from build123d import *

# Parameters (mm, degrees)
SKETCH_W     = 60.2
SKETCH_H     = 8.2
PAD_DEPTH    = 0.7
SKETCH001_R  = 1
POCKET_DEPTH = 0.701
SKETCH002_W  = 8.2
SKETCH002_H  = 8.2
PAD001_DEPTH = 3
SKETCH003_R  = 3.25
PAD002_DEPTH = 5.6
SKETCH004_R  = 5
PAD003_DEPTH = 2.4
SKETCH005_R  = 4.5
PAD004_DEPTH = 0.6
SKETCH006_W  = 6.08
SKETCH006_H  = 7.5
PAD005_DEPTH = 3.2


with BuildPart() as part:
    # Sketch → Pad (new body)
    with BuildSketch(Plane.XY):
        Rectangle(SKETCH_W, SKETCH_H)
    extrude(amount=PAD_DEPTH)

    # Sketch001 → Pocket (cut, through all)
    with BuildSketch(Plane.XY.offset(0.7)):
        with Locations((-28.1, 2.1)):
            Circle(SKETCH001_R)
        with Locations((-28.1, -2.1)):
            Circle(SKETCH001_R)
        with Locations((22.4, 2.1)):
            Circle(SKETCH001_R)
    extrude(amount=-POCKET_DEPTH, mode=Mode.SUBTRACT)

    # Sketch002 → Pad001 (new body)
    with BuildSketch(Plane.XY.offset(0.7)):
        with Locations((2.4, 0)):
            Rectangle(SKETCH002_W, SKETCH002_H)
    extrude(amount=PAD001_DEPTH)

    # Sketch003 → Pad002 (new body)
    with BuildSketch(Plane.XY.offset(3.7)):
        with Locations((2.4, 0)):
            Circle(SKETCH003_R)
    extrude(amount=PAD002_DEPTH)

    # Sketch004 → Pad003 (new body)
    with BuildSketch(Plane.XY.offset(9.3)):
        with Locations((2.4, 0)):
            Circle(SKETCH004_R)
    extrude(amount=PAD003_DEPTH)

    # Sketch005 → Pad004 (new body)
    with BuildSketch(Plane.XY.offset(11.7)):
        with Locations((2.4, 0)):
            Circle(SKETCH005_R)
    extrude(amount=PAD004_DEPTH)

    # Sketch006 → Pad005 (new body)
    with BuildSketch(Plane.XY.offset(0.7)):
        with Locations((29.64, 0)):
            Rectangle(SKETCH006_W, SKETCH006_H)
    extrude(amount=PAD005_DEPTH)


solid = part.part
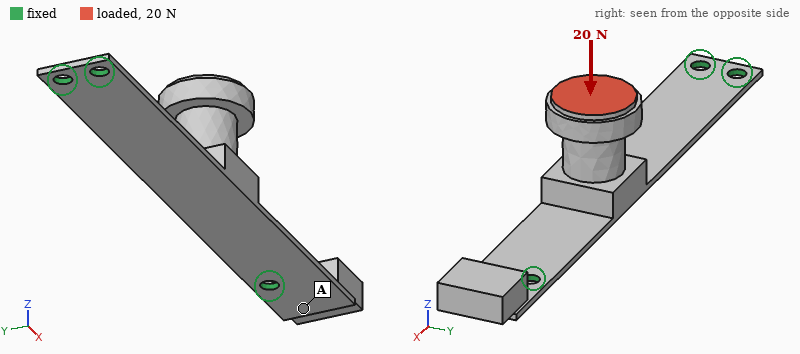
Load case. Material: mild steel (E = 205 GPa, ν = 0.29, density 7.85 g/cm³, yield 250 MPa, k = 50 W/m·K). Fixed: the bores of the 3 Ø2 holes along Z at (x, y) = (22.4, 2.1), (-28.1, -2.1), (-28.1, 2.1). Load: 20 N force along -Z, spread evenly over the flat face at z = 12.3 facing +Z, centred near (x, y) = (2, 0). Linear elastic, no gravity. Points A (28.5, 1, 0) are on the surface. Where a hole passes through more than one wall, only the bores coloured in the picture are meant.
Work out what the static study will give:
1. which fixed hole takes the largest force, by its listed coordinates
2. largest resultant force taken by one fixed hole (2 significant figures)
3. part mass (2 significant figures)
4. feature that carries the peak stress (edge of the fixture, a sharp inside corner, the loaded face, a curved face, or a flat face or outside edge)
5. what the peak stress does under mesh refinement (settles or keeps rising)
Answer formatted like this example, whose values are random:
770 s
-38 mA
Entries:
(22.4, 2.1)
15 N
8.6 g
edge of the fixture
keeps rising
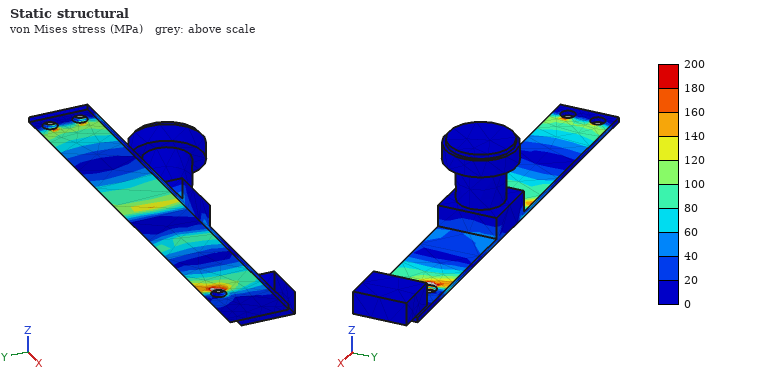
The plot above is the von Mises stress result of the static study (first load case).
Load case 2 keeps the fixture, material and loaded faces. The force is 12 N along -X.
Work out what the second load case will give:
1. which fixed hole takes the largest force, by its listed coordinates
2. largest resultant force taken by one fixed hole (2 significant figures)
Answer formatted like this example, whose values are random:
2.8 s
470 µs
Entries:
(22.4, 2.1)
7.1 N
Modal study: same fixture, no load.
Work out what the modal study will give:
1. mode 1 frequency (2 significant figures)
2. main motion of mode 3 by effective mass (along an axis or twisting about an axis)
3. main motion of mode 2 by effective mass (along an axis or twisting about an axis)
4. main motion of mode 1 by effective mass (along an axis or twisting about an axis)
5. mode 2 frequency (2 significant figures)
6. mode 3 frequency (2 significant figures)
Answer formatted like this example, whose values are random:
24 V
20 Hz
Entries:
760 Hz
along X
along Y
along Z
860 Hz
1800 Hz
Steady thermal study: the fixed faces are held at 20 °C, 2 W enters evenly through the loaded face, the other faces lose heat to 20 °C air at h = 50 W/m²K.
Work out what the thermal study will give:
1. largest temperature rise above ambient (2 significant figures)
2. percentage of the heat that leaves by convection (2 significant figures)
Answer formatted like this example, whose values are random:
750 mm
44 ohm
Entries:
40 K
67 %
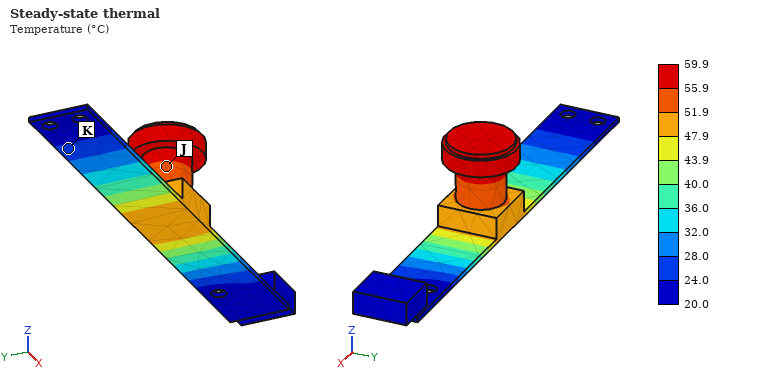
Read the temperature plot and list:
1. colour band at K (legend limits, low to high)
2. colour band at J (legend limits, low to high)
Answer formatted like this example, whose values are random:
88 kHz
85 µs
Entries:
24.0 to 28.0 °C
51.9 to 55.9 °C
